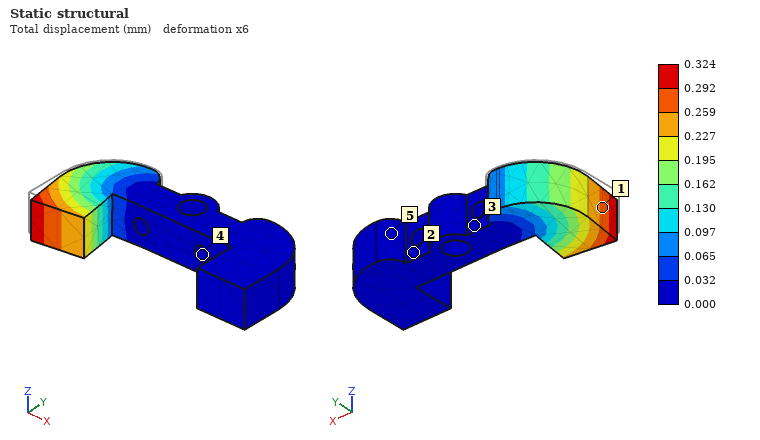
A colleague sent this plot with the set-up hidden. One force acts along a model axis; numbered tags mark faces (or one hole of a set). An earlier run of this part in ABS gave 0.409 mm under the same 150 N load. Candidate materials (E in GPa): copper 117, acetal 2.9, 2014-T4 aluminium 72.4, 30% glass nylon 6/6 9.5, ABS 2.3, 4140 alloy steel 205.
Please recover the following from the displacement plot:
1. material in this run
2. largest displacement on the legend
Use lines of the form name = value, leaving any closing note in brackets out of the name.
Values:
material in this run = acetal
largest displacement on the legend = 0.324 mm
